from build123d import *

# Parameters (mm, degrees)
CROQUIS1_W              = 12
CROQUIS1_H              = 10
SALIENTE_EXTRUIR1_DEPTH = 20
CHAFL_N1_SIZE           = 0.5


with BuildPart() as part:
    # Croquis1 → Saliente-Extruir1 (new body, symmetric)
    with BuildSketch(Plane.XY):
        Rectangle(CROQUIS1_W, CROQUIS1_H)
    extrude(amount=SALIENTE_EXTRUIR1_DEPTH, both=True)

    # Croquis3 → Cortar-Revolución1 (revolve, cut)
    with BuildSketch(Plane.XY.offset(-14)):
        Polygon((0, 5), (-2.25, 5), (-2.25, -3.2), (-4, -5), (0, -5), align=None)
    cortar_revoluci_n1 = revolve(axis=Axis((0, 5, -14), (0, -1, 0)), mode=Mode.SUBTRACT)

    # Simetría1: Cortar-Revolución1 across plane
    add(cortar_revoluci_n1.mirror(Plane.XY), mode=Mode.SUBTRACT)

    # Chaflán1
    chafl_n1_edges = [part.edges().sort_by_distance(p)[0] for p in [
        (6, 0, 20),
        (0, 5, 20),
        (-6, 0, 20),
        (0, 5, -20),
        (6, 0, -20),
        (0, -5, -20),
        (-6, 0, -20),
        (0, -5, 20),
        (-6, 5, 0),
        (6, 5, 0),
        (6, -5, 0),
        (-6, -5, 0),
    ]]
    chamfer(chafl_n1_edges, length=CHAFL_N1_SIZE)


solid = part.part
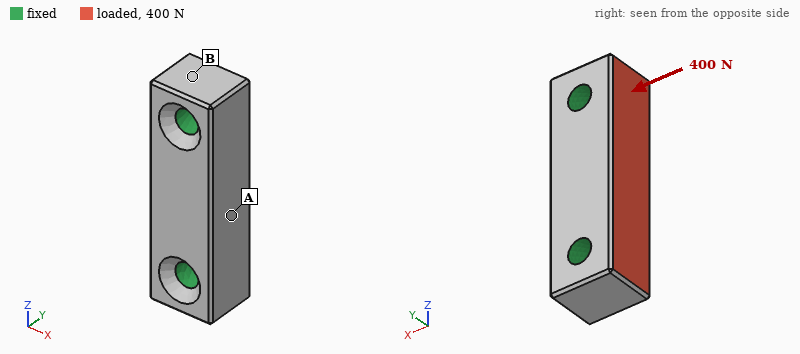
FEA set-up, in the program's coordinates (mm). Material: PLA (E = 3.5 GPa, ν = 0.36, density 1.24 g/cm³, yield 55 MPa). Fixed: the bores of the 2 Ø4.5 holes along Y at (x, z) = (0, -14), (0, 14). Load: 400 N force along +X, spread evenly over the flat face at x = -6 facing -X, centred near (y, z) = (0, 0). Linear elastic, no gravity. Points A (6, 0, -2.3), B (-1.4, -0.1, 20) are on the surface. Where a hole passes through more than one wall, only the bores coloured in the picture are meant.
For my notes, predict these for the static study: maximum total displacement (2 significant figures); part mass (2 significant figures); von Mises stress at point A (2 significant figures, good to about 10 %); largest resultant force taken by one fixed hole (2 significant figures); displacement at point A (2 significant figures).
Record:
13 µm
5.5 g
1.9 MPa
200 N
9.9 µm
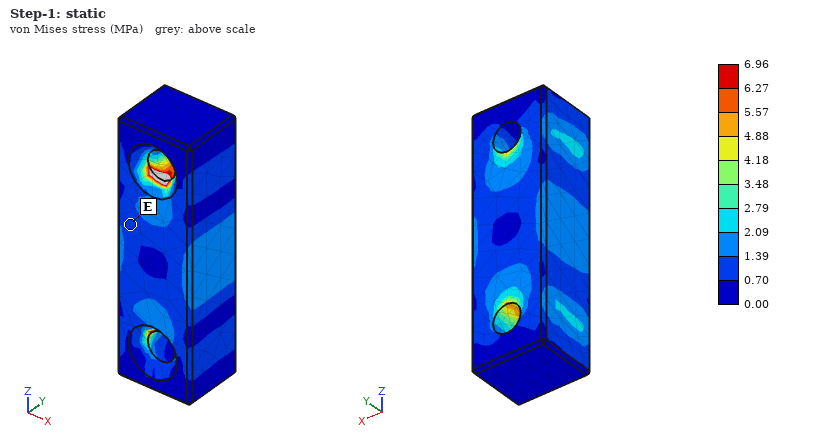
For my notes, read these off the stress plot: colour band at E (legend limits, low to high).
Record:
0.70 to 1.39 MPa
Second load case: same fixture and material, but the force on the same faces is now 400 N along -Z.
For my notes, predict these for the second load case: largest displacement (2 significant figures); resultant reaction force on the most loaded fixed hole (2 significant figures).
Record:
9.1 µm
210 N
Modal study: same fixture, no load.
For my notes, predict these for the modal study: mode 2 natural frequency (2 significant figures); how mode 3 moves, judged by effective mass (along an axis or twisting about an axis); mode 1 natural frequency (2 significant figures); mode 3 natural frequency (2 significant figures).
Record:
14 kHz
twisting about Z
13 kHz
16 kHz
